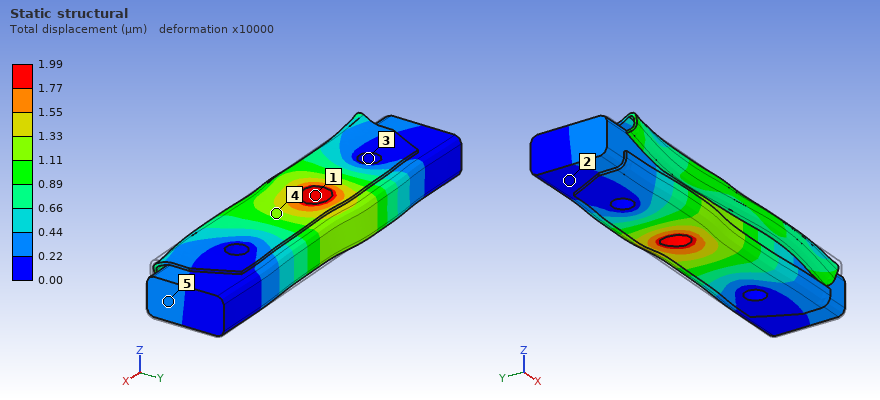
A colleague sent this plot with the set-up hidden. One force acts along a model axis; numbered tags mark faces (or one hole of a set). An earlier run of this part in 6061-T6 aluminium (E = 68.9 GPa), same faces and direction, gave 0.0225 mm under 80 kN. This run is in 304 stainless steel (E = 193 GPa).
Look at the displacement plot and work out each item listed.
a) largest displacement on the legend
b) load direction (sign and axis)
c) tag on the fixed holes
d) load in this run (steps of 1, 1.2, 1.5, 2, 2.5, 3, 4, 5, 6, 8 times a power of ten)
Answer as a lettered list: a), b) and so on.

a) 1.99 µm
b) -X
c) 3
d) 20 kN
